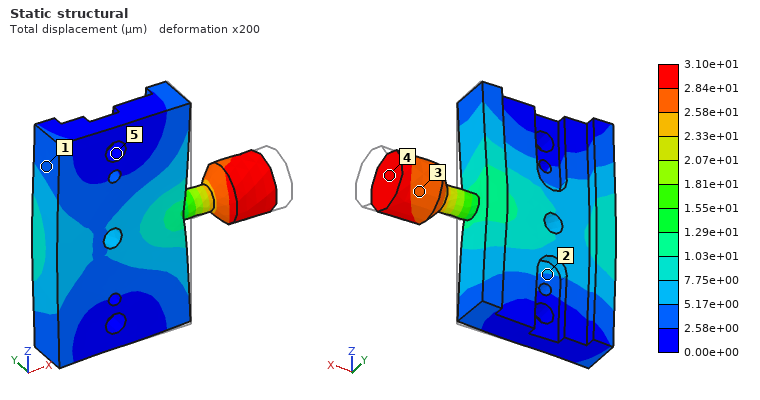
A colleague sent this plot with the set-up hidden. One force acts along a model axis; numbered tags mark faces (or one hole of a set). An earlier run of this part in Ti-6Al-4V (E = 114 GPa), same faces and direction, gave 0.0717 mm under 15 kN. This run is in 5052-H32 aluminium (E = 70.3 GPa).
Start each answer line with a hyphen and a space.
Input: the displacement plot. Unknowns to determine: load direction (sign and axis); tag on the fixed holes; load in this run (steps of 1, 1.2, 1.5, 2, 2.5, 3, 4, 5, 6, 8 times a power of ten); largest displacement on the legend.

- -X
- 5
- 4 kN
- 3.10e+01 µm
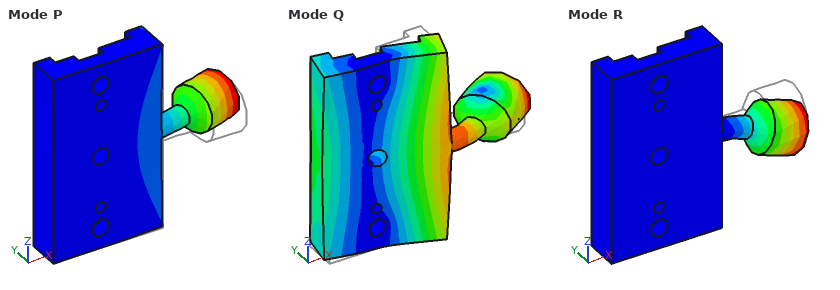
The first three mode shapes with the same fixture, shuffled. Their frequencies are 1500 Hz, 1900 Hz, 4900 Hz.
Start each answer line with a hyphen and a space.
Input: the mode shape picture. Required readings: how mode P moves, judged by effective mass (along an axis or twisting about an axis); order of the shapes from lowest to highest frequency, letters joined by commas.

- along Y
- P, R, Q
